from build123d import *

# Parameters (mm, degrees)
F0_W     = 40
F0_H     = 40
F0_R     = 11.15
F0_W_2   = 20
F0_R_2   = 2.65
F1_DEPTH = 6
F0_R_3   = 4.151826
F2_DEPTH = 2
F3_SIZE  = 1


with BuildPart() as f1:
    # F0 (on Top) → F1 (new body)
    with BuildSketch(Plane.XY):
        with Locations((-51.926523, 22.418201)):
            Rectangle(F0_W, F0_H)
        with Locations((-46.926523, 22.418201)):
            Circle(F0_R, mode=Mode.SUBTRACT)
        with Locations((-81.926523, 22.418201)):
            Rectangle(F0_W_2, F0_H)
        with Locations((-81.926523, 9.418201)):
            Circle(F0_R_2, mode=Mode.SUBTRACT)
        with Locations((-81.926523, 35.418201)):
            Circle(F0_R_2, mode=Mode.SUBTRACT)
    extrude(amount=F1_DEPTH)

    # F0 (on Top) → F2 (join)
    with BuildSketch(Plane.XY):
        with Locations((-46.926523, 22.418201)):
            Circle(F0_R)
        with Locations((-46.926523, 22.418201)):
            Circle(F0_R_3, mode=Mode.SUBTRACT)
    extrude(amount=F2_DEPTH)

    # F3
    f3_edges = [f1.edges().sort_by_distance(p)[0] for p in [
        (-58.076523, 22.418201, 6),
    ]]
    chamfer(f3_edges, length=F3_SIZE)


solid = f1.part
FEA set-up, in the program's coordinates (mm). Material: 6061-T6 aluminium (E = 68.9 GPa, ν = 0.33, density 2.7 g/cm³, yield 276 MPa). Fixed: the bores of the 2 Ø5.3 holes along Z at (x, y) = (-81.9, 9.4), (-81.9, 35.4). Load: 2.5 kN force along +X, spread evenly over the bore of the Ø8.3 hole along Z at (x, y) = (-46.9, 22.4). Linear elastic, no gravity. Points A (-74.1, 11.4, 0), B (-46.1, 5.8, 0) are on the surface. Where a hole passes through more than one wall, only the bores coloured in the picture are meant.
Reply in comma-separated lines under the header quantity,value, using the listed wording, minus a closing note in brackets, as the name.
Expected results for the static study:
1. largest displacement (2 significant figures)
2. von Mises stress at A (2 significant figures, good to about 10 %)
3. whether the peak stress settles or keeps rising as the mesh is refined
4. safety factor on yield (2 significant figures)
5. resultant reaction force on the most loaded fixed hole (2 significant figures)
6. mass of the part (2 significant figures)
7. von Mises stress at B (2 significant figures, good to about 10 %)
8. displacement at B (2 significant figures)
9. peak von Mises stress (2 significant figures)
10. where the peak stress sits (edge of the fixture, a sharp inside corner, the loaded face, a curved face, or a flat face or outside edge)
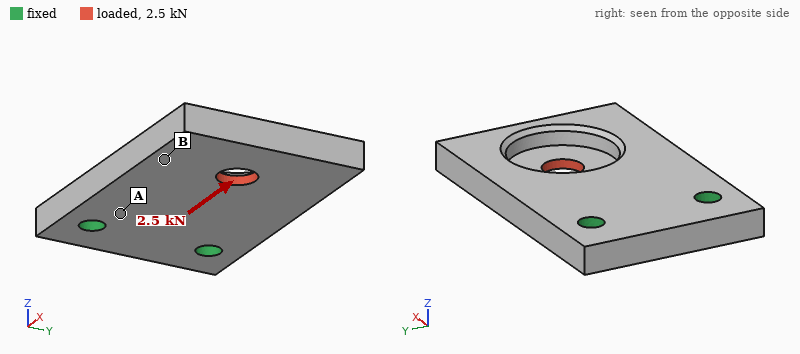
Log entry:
quantity,value
largest displacement,0.11 mm
von Mises stress at A,35 MPa
whether the peak stress settles or keeps rising as the mesh is refined,settles
safety factor on yield,2.7
resultant reaction force on the most loaded fixed hole,1.3 kN
mass of the part,34 g
von Mises stress at B,13 MPa
displacement at B,0.059 mm
peak von Mises stress,100 MPa
where the peak stress sits,the loaded face
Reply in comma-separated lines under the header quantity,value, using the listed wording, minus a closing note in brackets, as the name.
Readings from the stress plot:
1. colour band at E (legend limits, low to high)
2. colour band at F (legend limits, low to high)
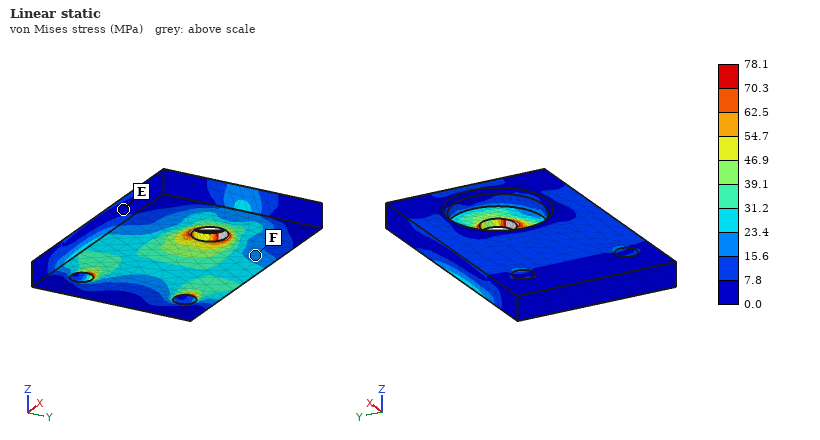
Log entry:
quantity,value
colour band at E,0.0 to 7.8 MPa
colour band at F,15.6 to 23.4 MPa
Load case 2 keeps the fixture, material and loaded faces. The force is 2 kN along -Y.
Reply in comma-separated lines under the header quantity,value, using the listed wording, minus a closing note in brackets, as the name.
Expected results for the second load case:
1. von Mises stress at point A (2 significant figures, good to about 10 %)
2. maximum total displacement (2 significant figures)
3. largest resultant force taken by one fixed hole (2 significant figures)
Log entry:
quantity,value
von Mises stress at point A,30 MPa
maximum total displacement,53 µm
largest resultant force taken by one fixed hole,2.6 kN
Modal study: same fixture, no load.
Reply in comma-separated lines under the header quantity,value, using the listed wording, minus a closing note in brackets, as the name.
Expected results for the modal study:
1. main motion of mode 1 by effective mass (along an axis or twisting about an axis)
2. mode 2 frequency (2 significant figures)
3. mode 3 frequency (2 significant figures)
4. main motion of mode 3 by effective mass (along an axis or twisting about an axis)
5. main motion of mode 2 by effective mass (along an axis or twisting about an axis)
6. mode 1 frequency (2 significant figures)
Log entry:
quantity,value
main motion of mode 1 by effective mass,along Z
mode 2 frequency,4900 Hz
mode 3 frequency,9400 Hz
main motion of mode 3 by effective mass,along Y
main motion of mode 2 by effective mass,twisting about X
mode 1 frequency,2200 Hz
